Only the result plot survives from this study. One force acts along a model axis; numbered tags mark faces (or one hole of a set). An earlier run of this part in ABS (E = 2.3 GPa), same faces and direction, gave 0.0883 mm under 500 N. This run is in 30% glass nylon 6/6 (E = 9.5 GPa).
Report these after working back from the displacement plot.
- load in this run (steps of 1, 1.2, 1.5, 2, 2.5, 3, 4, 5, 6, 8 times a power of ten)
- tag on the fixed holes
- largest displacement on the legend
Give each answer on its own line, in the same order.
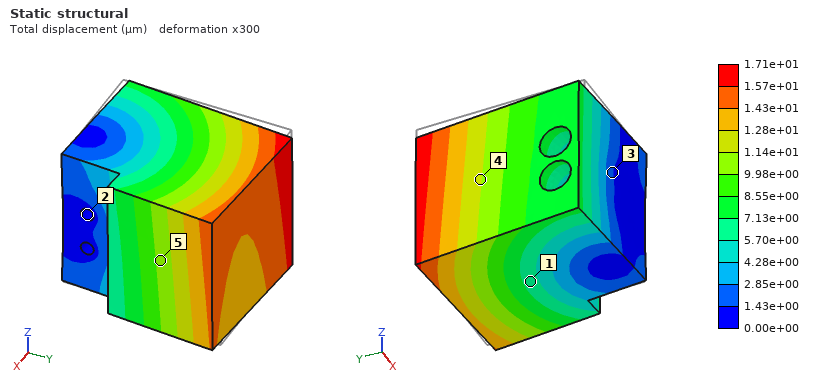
400 N
2
1.71e+01 µm
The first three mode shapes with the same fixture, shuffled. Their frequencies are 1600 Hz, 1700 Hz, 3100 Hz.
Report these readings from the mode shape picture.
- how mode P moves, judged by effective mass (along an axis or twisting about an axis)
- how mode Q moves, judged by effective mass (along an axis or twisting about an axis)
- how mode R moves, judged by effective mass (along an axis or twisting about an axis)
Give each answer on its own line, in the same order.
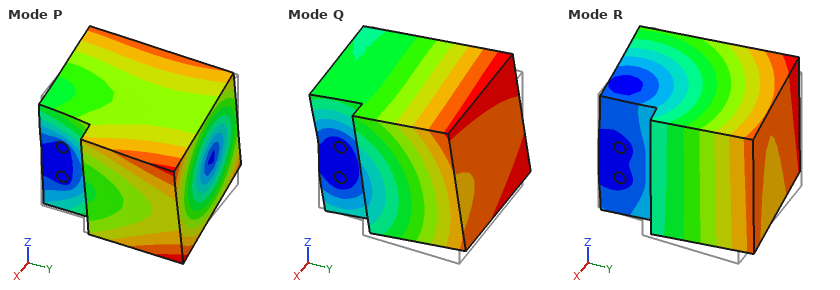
twisting about Y
along Z
along X
